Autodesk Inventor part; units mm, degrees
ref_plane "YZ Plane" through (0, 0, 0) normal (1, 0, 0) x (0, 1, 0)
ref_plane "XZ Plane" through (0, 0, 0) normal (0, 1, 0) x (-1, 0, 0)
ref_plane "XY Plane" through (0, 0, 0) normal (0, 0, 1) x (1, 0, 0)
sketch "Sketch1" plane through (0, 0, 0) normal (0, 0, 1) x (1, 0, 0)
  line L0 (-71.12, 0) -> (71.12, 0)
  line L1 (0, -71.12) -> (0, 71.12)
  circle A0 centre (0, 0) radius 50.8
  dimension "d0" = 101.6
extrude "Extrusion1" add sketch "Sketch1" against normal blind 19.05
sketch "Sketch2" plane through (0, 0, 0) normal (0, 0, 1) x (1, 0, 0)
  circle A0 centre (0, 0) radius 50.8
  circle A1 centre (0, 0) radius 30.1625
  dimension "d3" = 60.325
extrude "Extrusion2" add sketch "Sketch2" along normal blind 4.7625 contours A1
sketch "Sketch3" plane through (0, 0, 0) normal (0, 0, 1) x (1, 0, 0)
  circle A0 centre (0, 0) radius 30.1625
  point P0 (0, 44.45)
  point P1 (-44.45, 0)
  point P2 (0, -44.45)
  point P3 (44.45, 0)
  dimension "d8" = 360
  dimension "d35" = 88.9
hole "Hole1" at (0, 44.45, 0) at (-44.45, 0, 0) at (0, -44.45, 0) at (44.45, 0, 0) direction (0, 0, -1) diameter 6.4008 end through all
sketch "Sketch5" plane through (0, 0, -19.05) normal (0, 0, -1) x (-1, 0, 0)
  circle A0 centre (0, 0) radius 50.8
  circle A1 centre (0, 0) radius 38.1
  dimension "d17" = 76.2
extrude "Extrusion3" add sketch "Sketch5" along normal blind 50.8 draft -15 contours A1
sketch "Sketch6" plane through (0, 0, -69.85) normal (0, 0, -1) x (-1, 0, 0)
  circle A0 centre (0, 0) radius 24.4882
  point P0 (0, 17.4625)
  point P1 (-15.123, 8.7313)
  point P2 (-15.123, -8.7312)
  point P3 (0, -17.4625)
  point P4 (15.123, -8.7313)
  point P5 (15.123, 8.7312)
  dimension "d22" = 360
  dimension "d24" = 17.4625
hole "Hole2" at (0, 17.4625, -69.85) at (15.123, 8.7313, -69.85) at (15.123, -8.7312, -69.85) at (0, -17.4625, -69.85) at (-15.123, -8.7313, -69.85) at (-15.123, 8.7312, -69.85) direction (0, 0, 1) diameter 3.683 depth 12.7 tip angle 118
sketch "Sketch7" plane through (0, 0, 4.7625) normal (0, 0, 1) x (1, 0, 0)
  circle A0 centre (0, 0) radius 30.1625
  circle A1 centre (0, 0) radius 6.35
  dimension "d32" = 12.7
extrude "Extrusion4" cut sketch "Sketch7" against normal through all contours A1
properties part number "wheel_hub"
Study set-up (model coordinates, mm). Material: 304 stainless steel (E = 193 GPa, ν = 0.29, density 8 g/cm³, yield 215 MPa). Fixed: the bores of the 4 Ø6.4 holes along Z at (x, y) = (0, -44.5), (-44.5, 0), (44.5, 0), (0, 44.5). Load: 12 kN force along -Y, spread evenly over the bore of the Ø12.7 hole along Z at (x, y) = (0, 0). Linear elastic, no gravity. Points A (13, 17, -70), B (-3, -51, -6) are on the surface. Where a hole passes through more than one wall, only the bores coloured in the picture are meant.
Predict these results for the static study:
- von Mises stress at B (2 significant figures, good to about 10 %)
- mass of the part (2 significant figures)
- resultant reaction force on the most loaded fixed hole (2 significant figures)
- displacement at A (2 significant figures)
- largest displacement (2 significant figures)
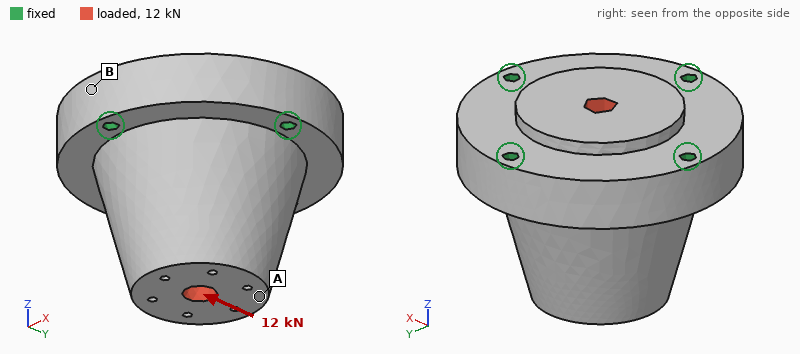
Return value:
6.8 MPa
2.5 kg
5.0 kN
4.2 µm
4.4 µm
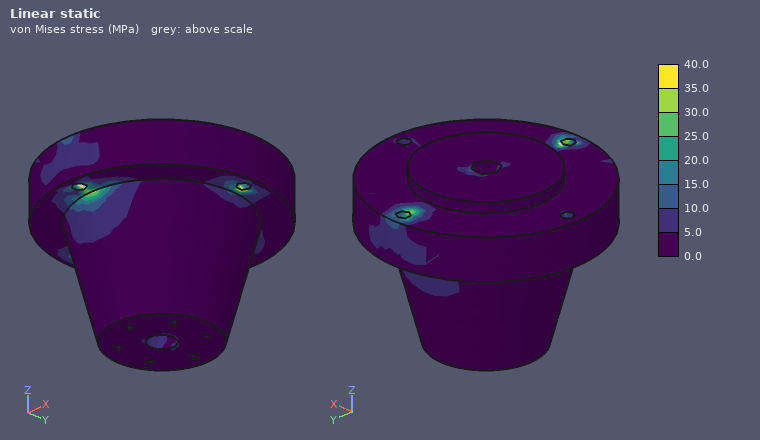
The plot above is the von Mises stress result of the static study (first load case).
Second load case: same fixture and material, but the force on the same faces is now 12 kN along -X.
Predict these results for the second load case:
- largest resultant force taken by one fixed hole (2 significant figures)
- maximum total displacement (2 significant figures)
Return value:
5.0 kN
4.4 µm
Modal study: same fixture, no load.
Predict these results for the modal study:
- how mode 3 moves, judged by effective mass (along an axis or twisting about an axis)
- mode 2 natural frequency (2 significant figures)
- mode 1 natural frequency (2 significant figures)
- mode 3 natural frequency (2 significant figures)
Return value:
along Z
7800 Hz
7800 Hz
9500 Hz
